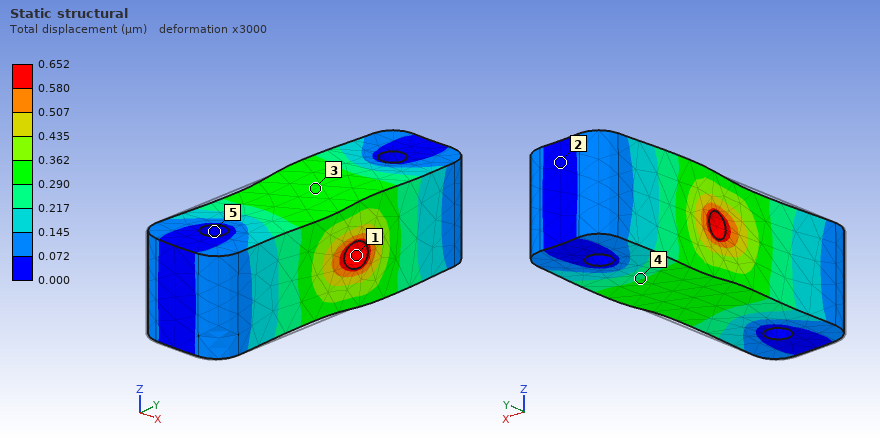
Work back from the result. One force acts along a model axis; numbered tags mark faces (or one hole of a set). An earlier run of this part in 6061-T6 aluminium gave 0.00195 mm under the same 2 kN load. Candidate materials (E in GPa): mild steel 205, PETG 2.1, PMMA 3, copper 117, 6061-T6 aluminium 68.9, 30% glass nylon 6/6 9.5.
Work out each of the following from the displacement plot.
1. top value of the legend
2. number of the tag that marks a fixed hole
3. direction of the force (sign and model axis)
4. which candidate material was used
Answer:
0.652 µm
5
+Y
mild steel
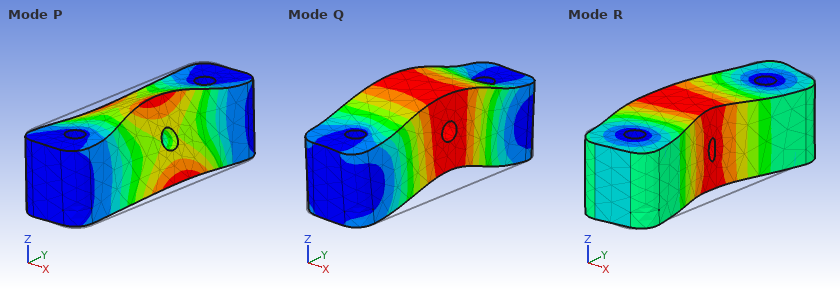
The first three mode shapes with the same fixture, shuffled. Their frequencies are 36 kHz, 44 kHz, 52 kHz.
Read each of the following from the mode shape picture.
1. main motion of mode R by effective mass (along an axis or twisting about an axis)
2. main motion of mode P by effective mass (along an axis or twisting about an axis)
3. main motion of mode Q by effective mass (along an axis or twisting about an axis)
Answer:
along X
twisting about Y
along Z
